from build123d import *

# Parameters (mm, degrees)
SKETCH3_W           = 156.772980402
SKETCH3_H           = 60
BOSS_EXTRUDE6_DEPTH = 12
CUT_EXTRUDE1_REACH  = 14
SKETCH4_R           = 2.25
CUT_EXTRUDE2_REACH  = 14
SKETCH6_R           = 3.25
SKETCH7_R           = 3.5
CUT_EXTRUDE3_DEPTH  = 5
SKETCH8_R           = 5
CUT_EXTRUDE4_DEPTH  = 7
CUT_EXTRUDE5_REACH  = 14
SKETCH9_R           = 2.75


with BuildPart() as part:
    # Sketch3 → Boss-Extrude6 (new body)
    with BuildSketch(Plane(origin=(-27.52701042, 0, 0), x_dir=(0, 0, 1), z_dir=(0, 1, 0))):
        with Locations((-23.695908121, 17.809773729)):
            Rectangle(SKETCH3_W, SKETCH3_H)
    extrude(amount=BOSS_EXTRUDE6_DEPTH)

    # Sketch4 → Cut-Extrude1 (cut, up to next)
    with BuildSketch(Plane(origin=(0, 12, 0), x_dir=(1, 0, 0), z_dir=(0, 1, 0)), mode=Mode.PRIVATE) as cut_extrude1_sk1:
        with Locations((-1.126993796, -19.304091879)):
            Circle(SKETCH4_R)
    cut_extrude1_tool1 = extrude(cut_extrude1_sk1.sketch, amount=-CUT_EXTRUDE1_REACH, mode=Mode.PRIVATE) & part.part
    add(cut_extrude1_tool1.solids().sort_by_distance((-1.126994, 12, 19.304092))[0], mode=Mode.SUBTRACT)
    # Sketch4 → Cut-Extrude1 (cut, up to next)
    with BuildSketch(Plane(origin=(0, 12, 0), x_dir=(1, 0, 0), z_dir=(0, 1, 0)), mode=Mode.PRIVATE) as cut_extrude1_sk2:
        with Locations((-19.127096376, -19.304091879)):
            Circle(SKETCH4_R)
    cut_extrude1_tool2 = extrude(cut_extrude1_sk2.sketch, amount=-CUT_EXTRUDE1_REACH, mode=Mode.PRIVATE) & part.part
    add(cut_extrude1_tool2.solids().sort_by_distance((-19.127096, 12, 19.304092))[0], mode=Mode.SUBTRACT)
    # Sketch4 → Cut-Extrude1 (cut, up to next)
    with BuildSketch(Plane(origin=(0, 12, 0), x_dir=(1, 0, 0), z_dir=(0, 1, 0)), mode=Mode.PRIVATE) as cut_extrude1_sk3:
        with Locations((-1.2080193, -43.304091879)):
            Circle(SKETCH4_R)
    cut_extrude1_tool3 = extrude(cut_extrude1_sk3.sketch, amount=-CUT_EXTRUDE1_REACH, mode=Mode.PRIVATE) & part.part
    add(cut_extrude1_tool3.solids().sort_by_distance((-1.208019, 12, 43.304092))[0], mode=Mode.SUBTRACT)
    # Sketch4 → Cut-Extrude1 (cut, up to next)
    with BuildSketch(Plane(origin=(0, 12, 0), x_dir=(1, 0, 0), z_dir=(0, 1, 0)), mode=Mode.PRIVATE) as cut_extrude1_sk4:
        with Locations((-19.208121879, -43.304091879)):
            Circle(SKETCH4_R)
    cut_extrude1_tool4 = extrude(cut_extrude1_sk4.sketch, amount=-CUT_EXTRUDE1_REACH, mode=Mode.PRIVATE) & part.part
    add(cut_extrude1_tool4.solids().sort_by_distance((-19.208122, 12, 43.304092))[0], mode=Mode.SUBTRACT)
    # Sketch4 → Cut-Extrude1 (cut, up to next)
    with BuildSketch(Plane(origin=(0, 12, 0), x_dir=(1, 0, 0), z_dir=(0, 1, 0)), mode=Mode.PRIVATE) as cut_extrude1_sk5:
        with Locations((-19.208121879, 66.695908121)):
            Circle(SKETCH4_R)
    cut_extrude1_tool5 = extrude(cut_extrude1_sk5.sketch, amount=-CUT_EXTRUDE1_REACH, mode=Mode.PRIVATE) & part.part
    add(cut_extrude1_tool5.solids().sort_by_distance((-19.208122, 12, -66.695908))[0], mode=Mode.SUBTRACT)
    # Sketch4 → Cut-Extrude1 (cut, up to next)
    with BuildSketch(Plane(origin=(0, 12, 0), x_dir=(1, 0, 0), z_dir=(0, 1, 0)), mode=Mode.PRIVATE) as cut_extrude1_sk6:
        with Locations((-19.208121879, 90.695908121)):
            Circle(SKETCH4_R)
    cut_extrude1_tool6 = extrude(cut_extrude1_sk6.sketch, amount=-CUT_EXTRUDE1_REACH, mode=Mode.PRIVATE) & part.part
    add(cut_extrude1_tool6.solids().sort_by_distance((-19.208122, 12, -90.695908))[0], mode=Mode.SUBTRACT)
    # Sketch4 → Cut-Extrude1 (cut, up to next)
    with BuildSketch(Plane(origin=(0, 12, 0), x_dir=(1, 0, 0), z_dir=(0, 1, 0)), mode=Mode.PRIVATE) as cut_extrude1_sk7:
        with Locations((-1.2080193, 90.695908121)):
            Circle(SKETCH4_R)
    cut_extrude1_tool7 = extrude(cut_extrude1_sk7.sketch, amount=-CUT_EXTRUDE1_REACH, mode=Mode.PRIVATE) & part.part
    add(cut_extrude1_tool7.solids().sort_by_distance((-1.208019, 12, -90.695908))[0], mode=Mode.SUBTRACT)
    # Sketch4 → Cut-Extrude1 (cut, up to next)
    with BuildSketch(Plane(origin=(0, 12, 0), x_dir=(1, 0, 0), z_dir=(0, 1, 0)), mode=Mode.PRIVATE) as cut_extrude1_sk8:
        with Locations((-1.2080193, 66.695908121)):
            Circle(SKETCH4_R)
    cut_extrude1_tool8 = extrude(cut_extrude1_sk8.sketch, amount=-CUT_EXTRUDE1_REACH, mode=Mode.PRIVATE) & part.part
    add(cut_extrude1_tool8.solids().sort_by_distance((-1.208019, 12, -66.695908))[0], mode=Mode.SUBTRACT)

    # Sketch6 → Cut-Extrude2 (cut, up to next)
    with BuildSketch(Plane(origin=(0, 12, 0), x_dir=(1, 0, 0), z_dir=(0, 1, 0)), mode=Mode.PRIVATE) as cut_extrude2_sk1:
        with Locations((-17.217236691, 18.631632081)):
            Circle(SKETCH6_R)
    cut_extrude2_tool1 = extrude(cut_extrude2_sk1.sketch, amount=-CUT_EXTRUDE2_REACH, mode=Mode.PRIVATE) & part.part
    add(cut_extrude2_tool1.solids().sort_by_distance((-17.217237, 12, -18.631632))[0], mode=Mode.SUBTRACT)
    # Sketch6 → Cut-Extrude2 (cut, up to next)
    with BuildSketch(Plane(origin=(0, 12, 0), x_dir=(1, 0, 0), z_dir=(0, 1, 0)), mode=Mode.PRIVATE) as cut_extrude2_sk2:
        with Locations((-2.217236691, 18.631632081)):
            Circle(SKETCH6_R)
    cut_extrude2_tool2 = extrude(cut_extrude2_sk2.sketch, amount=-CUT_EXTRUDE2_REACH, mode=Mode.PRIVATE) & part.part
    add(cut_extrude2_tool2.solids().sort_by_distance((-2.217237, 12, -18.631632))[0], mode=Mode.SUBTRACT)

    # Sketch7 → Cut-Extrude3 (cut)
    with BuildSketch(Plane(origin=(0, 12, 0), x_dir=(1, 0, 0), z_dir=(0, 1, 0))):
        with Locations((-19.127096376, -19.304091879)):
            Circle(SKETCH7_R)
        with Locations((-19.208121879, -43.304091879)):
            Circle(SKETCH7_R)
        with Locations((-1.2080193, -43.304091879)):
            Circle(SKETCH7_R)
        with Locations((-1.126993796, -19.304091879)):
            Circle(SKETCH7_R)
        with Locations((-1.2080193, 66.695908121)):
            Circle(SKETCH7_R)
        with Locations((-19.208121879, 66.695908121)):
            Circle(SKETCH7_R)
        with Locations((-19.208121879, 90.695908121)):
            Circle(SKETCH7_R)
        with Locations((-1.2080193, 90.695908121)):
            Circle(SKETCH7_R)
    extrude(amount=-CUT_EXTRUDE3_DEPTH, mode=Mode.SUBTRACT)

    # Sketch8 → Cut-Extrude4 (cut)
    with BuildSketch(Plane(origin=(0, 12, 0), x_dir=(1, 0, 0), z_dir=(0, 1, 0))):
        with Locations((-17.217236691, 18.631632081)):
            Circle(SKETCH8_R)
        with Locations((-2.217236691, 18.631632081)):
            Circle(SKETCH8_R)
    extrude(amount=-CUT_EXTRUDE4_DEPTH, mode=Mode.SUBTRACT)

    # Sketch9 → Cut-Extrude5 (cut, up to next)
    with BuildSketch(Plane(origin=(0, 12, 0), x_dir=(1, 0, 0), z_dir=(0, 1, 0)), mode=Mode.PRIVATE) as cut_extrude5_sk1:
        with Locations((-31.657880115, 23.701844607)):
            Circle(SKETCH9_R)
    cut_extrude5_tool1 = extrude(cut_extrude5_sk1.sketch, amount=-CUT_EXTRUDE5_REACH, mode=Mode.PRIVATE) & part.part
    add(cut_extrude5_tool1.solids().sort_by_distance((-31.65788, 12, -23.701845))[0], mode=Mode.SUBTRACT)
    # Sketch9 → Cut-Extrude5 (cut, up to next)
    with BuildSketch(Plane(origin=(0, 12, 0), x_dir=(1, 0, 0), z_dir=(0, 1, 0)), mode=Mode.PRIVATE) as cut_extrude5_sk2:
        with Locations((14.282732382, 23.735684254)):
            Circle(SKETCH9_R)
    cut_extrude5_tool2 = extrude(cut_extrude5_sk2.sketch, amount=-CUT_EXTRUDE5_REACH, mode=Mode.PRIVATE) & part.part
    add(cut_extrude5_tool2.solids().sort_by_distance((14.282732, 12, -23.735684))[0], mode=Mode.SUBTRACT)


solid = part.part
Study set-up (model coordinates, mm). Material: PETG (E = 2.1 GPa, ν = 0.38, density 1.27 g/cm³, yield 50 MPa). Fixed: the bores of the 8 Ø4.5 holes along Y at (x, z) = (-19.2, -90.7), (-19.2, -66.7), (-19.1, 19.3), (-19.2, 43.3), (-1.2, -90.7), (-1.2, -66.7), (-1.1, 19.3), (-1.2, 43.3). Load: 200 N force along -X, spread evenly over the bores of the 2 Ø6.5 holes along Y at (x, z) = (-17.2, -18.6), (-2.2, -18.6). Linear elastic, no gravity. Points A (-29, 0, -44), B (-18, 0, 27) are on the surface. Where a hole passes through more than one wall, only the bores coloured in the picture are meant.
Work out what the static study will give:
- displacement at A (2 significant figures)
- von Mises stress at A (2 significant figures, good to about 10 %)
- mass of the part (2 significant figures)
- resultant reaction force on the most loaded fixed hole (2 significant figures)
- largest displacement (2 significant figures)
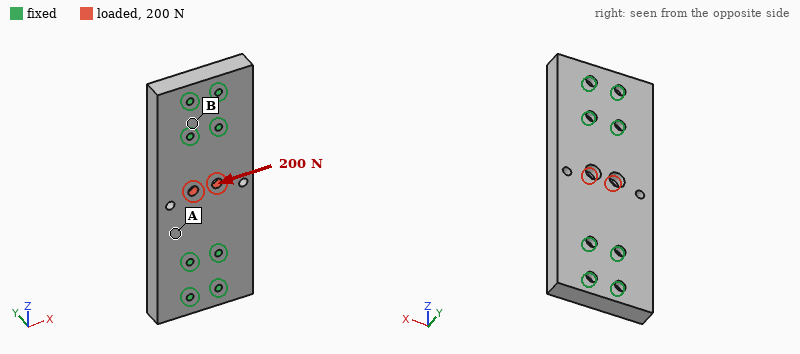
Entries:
9.5 µm
0.34 MPa
140 g
71 N
20 µm
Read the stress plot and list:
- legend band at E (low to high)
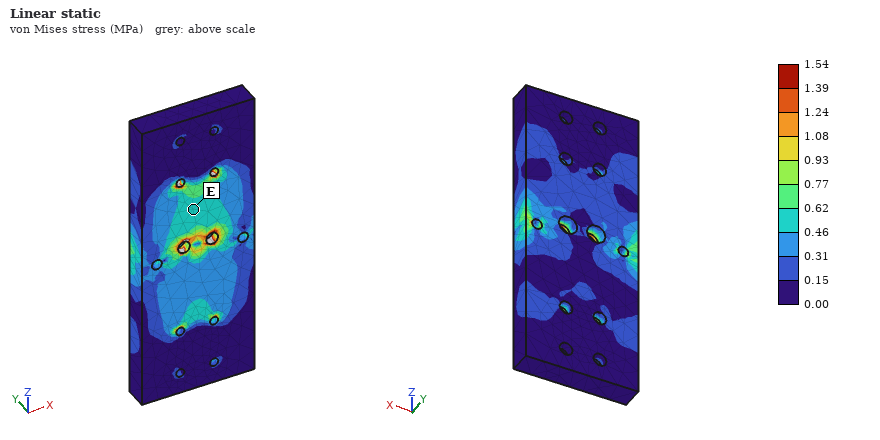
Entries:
0.46 to 0.62 MPa
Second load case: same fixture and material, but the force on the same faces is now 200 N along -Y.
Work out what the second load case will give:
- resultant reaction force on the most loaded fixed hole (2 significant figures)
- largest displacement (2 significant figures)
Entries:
93 N
78 µm
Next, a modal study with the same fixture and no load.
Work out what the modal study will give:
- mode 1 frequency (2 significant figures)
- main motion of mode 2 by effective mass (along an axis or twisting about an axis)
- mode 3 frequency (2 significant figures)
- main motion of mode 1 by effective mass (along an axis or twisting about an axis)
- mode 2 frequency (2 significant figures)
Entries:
1500 Hz
twisting about Z
3100 Hz
along Y
1700 Hz
